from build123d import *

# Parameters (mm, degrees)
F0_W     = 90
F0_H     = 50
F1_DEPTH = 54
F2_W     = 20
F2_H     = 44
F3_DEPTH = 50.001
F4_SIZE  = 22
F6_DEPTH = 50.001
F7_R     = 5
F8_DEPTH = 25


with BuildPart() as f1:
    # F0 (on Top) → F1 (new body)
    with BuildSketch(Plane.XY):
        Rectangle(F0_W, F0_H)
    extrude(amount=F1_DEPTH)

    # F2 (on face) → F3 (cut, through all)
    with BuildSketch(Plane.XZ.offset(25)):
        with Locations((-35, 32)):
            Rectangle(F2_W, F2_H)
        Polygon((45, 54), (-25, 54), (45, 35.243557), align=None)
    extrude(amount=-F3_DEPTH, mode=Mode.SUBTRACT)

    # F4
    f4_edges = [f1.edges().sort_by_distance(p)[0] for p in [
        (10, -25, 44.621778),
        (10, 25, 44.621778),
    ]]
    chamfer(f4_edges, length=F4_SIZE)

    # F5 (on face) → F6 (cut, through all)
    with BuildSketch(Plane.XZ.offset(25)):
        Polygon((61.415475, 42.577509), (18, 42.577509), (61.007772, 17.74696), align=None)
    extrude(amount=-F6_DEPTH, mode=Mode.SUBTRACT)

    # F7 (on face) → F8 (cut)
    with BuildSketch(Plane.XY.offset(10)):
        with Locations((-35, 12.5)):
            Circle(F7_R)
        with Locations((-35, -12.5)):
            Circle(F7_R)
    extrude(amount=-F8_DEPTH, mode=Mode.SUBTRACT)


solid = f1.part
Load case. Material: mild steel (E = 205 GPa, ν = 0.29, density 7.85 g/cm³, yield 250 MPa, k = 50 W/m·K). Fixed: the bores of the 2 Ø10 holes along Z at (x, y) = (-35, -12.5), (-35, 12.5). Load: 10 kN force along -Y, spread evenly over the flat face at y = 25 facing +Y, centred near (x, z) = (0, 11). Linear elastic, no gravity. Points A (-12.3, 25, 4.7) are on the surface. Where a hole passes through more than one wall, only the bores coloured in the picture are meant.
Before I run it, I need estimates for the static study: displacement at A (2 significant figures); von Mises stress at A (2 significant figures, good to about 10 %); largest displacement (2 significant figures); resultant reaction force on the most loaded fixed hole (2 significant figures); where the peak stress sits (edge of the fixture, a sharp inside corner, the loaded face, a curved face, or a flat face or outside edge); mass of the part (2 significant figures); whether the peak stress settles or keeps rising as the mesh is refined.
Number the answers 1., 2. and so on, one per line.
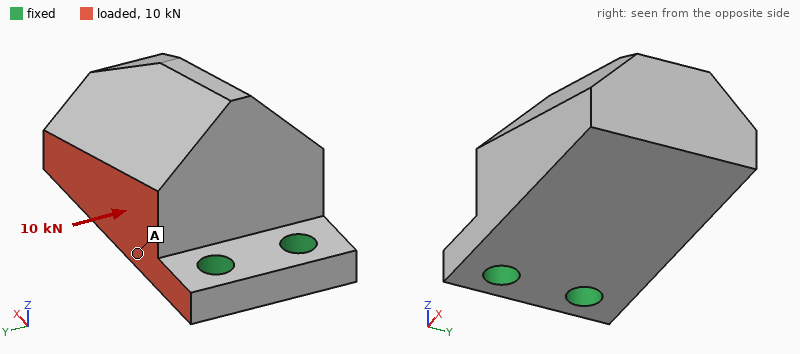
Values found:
1. 11 µm
2. 23 MPa
3. 32 µm
4. 12 kN
5. edge of the fixture
6. 1.0 kg
7. keeps rising
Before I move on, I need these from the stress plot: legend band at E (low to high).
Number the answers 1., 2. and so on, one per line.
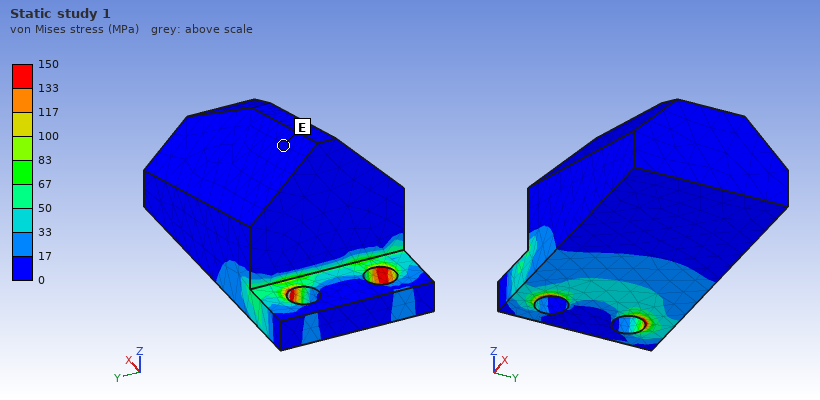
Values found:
1. 0 to 17 MPa
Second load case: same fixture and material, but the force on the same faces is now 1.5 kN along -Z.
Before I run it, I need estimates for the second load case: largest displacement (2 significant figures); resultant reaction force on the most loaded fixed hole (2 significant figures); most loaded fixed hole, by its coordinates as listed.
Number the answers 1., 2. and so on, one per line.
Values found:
1. 48 µm
2. 1.8 kN
3. (-35, 12.5)
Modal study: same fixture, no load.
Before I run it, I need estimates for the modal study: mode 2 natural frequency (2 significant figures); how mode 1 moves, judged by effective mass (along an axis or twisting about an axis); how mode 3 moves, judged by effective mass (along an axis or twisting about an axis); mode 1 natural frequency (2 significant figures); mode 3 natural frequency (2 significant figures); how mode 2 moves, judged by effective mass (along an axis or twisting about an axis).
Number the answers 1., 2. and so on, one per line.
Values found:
1. 3300 Hz
2. along Z
3. twisting about X
4. 1000 Hz
5. 4700 Hz
6. along Y
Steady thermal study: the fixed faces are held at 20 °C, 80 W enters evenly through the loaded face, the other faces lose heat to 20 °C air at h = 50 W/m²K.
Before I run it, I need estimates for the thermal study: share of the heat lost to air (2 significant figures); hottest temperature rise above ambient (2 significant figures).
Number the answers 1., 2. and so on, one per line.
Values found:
1. 29 %
2. 54 K
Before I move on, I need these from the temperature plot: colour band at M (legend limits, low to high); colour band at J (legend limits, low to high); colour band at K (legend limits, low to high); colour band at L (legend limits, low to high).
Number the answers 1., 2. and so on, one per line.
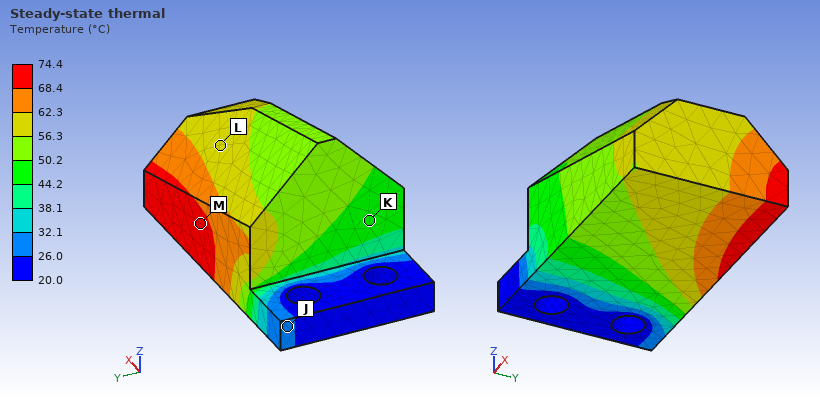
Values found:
1. 68.4 to 74.4 °C
2. 26.0 to 32.1 °C
3. 44.2 to 50.2 °C
4. 56.3 to 62.3 °C
